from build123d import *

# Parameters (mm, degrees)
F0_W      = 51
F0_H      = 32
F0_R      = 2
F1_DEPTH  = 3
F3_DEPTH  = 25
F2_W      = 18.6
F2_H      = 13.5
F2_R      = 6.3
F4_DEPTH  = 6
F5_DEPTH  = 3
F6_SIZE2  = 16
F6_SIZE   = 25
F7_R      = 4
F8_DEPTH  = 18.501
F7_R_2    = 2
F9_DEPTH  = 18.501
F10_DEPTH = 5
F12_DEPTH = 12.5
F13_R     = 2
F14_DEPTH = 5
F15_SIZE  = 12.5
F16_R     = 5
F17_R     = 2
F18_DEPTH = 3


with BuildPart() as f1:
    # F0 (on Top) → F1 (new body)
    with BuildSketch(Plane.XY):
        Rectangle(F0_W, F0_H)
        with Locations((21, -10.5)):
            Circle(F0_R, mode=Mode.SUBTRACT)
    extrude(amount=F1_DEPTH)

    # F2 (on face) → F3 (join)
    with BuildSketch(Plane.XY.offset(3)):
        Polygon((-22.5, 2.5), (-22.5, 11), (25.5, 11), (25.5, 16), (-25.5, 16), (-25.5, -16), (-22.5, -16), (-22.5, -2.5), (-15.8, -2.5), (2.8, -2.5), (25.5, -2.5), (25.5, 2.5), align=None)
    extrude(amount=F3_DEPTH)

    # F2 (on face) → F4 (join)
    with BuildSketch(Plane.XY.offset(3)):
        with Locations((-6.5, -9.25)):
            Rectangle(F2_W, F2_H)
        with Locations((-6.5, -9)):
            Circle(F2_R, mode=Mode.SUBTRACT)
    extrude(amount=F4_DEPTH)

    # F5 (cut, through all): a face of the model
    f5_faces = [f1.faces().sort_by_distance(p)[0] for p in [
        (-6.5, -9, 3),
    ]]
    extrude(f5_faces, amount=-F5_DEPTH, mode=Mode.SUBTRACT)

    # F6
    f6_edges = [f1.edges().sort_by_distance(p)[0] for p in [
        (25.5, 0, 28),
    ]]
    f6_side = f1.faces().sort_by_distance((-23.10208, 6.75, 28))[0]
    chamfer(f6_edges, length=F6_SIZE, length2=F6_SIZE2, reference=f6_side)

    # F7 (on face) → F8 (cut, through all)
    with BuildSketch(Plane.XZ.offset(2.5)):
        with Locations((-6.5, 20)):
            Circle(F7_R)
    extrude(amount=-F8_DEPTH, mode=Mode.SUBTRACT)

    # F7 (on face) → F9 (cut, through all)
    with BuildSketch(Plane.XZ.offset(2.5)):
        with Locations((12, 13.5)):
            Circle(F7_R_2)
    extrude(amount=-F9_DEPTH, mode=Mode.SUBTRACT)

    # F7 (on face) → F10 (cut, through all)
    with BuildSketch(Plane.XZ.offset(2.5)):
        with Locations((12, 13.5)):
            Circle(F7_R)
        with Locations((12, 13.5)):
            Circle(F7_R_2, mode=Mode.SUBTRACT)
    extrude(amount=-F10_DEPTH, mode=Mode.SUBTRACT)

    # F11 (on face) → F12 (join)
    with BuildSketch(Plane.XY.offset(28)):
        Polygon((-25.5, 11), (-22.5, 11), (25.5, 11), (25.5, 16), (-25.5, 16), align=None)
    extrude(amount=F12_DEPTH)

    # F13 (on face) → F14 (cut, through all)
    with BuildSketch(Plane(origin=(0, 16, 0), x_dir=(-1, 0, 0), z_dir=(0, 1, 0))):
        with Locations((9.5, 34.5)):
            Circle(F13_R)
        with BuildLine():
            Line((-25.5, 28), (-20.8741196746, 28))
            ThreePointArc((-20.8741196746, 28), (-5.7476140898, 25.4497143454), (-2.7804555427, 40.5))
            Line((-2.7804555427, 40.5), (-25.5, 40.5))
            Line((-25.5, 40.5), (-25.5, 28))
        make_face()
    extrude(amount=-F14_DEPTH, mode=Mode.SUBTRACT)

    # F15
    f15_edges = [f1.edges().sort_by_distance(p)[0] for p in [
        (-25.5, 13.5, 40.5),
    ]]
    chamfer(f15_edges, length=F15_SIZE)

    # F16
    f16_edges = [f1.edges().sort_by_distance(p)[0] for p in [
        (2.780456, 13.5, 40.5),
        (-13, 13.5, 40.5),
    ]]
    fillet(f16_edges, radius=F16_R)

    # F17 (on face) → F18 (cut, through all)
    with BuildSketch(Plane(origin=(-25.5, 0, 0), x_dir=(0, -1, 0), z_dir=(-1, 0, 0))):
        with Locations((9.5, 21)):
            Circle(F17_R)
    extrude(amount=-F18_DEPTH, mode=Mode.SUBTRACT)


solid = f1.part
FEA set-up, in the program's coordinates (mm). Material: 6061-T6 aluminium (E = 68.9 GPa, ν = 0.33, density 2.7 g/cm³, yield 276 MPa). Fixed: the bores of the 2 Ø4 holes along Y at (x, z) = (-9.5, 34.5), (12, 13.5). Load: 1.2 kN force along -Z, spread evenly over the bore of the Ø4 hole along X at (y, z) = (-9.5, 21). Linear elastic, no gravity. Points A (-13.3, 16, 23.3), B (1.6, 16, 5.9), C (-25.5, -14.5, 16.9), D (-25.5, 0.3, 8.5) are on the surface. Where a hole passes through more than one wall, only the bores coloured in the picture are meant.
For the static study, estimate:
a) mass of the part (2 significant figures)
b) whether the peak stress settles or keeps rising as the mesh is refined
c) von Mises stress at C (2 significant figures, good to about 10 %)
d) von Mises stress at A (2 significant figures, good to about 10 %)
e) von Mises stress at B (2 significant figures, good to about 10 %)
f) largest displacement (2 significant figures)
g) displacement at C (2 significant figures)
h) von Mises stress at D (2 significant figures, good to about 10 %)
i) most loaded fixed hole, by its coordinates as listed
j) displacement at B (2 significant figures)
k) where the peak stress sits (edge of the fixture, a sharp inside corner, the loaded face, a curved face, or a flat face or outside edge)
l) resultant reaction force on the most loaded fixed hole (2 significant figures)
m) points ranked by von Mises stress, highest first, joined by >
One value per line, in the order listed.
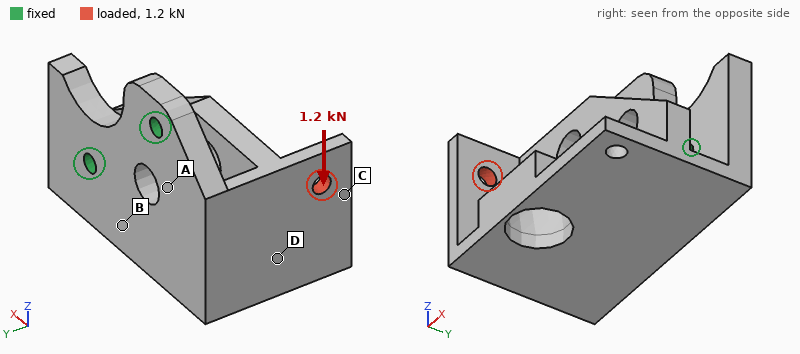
51 g
keeps rising
17 MPa
88 MPa
63 MPa
0.50 mm
0.41 mm
32 MPa
(-9.5, 34.5)
0.079 mm
edge of the fixture
1.5 kN
A > B > D > C
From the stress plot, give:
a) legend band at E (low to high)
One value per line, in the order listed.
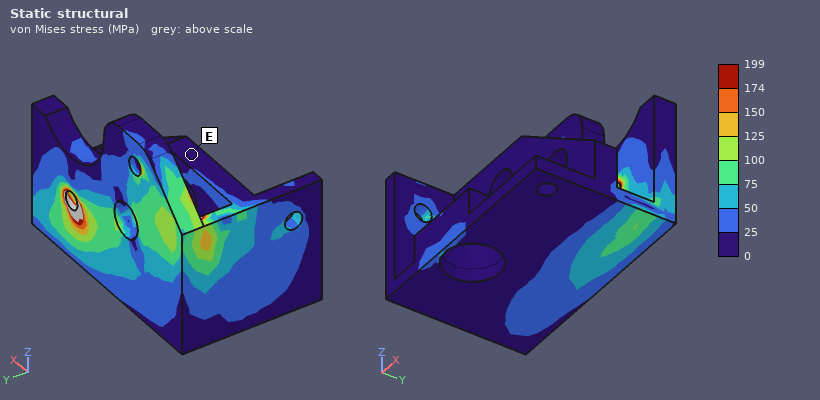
0 to 25 MPa
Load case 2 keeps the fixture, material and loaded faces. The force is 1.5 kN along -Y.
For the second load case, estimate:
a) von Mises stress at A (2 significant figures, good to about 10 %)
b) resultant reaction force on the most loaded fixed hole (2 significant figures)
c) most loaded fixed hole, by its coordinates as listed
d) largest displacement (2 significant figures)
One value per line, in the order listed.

66 MPa
1.3 kN
(-9.5, 34.5)
0.32 mm
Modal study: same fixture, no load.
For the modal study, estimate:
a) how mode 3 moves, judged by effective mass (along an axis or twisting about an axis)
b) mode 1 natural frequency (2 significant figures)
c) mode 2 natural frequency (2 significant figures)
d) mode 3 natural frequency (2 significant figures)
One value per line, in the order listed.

along Y
1900 Hz
3600 Hz
5200 Hz
